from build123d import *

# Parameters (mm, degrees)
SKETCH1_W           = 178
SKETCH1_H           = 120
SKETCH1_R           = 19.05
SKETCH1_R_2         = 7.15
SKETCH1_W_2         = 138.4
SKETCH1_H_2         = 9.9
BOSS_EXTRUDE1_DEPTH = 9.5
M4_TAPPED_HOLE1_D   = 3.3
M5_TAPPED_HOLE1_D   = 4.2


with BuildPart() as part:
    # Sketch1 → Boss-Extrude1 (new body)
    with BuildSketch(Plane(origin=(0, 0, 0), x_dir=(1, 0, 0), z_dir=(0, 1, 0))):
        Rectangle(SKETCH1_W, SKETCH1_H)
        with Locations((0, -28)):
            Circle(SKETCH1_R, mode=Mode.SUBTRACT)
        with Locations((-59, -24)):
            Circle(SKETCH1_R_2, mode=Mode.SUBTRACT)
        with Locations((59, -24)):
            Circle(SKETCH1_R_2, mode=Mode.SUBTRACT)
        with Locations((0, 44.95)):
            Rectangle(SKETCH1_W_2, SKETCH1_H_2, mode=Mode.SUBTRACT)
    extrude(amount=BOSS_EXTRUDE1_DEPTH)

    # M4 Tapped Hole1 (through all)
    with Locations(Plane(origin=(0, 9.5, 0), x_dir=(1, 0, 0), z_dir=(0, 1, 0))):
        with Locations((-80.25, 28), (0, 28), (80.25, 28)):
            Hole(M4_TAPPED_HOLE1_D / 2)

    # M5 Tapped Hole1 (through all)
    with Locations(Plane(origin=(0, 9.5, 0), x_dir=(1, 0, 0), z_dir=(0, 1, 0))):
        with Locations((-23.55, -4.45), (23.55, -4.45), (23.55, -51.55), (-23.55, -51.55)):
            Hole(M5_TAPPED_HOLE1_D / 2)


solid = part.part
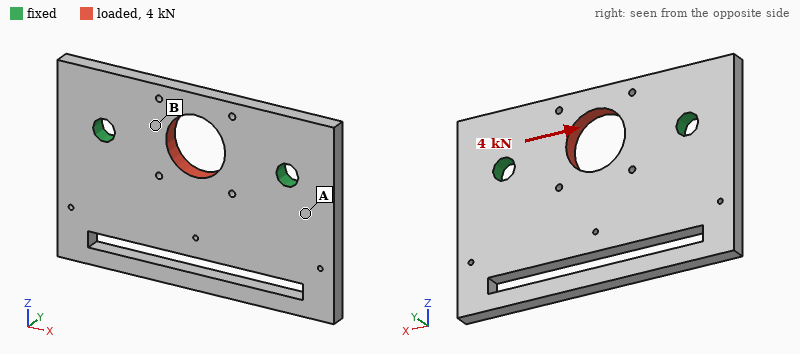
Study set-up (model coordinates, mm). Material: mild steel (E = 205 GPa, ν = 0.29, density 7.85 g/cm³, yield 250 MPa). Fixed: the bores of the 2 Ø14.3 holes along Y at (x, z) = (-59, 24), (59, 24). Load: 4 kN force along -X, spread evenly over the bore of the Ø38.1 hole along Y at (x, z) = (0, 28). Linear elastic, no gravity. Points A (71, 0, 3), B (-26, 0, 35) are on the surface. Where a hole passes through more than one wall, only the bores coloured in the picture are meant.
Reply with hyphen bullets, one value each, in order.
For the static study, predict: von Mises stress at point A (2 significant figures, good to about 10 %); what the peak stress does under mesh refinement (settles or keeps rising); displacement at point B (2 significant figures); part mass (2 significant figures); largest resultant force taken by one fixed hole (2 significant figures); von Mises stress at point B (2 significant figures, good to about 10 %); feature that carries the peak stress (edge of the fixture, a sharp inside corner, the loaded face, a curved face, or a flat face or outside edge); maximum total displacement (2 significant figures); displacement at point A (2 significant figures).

- 1.4 MPa
- keeps rising
- 0.82 µm
- 1.4 kg
- 2.0 kN
- 4.8 MPa
- edge of the fixture
- 1.4 µm
- 0.24 µm
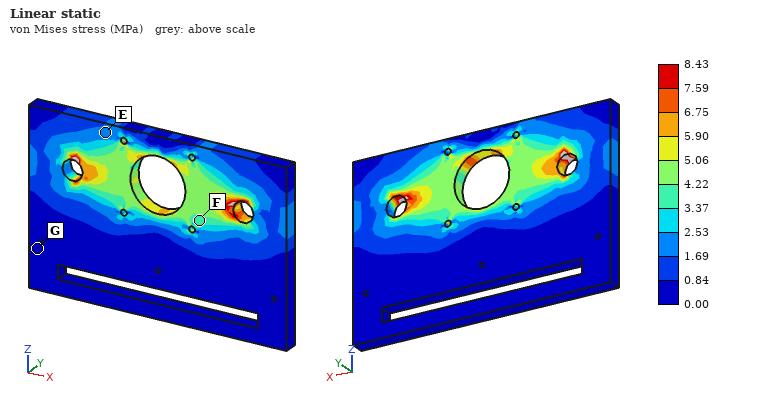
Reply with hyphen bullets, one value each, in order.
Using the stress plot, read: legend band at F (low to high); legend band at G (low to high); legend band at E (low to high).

- 3.37 to 4.22 MPa
- 0.00 to 0.84 MPa
- 1.69 to 2.53 MPa
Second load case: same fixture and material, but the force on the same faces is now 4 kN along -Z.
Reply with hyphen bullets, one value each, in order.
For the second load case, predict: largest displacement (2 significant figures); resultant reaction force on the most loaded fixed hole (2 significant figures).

- 3.4 µm
- 2.0 kN
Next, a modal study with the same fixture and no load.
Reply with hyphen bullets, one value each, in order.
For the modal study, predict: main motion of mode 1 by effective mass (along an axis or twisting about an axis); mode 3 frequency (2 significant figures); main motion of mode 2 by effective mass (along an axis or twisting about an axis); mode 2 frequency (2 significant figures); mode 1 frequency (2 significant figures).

- along Y
- 2100 Hz
- twisting about Z
- 1600 Hz
- 1000 Hz
